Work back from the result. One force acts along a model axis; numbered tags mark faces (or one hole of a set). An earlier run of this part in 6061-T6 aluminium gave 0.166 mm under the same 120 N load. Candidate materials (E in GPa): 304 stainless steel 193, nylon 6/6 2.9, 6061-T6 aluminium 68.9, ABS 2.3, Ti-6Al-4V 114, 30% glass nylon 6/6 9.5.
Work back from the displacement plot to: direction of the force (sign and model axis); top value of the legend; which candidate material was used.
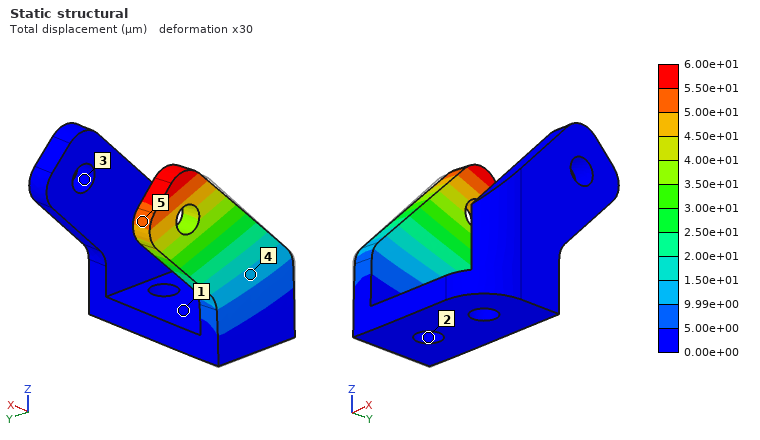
+X
6.00e+01 µm
304 stainless steel
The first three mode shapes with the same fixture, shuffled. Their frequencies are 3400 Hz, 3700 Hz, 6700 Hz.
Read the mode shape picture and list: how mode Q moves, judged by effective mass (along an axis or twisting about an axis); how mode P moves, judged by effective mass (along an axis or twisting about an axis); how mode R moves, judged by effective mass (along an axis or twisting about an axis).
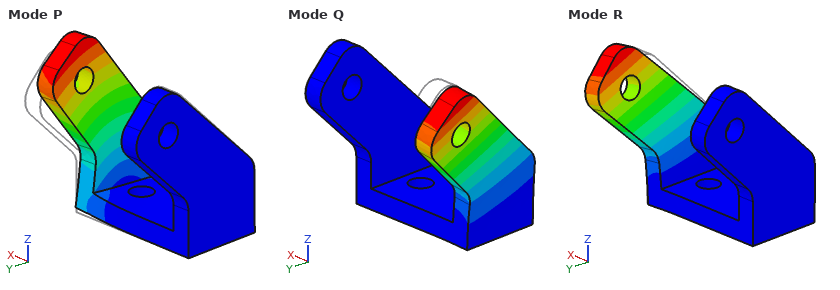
along X
along Y
along X
